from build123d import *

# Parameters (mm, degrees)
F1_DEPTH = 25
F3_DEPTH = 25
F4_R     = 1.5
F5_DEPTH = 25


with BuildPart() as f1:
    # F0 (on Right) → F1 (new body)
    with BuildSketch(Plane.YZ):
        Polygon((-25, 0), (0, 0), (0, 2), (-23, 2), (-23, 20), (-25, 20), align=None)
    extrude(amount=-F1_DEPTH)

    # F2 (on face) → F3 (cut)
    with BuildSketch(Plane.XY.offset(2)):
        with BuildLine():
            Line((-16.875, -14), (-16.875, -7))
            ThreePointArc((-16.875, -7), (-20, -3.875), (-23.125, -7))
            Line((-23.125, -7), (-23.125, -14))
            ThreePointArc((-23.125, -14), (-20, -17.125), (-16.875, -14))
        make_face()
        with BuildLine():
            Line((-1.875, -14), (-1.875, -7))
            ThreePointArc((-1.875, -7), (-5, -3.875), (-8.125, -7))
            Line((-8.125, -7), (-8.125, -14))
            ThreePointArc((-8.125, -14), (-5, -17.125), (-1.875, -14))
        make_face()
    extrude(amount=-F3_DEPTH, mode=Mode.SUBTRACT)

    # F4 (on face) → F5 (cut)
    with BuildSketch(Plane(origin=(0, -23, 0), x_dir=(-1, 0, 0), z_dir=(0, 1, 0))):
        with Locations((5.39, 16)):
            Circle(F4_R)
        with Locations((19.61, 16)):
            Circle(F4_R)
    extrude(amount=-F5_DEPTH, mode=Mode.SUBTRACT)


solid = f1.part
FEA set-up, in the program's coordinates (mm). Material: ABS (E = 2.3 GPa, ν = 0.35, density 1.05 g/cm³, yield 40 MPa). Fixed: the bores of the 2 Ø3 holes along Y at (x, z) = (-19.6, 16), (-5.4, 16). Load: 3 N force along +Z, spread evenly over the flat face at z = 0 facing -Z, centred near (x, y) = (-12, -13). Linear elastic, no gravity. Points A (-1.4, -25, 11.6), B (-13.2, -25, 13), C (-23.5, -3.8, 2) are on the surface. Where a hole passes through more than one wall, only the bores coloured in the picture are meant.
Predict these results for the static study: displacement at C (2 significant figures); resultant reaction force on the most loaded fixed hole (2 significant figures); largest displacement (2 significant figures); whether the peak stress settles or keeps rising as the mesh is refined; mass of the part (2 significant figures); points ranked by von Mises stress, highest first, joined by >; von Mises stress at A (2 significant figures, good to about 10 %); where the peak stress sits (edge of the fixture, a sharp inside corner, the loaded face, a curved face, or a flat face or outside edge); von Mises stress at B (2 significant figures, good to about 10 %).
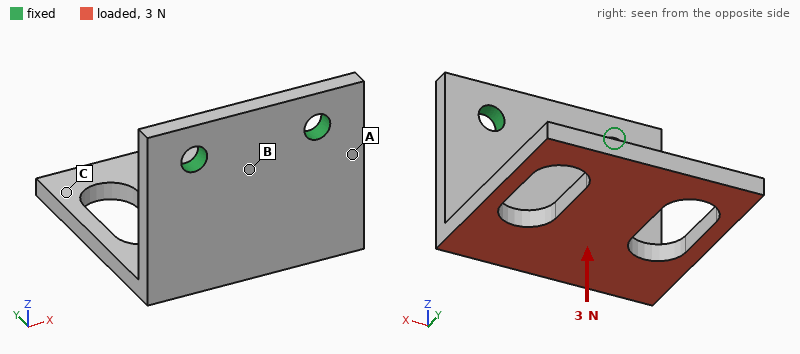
0.34 mm
1.6 N
0.43 mm
keeps rising
1.9 g
A > B > C
1.9 MPa
edge of the fixture
1.3 MPa
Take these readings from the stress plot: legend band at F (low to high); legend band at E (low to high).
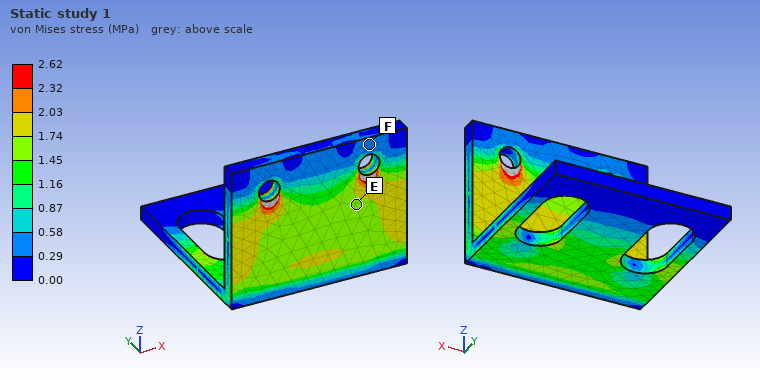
0.29 to 0.58 MPa
1.45 to 1.74 MPa
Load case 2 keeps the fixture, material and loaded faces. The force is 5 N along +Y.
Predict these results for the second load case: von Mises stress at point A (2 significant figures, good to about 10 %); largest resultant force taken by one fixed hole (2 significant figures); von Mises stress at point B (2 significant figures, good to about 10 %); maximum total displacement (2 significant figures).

3.4 MPa
2.5 N
2.6 MPa
0.41 mm
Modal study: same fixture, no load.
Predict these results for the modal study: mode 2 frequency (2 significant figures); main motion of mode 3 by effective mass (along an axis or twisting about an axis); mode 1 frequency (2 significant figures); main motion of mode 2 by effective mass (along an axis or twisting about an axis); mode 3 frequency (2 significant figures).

900 Hz
along Y
480 Hz
along X
1400 Hz
